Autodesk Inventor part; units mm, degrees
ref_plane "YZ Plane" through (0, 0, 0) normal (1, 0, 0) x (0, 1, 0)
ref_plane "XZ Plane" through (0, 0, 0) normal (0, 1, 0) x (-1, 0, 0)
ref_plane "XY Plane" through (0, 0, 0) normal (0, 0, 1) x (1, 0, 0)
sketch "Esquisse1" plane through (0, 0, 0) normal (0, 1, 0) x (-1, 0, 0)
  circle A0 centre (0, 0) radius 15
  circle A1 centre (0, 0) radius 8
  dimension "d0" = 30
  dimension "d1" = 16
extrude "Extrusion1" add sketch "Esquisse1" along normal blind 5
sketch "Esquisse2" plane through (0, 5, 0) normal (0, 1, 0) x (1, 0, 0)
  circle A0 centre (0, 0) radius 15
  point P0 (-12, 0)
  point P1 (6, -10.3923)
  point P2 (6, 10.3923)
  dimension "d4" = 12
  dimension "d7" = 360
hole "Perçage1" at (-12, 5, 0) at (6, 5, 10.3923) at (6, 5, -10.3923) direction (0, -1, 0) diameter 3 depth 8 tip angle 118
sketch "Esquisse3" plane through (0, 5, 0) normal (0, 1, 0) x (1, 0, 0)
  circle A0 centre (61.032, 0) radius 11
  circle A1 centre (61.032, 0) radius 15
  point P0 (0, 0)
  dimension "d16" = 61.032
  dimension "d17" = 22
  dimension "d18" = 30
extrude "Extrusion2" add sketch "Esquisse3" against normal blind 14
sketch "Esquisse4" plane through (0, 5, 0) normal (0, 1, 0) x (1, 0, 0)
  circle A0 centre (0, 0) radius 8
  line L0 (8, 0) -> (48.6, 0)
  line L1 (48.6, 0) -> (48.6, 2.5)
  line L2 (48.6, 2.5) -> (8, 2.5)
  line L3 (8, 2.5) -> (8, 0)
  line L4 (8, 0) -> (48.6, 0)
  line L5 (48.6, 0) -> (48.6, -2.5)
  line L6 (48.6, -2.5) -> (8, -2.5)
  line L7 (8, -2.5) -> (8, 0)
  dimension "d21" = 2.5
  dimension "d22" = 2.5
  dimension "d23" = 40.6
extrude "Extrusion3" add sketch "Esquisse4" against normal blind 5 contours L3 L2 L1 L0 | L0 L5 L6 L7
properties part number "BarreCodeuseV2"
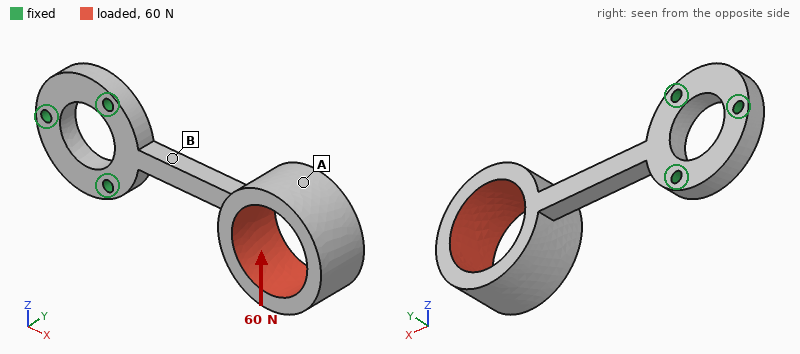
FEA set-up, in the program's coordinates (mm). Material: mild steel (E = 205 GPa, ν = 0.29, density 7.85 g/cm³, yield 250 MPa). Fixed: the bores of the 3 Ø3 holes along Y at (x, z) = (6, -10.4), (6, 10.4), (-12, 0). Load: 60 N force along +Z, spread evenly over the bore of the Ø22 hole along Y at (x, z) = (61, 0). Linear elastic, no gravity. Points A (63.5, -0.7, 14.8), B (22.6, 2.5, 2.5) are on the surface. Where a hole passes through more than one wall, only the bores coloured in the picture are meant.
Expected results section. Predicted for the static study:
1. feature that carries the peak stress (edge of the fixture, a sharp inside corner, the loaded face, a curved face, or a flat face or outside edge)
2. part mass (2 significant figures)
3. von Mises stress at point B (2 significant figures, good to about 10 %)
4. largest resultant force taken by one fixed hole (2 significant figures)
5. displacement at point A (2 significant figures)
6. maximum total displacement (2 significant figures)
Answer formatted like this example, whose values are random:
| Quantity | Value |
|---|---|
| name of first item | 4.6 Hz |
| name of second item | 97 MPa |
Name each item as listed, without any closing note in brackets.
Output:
| Quantity | Value |
|---|---|
| feature that carries the peak stress | a flat face or outside edge |
| part mass | 61 g |
| von Mises stress at point B | 110 MPa |
| largest resultant force taken by one fixed hole | 200 N |
| displacement at point A | 0.25 mm |
| maximum total displacement | 0.32 mm |
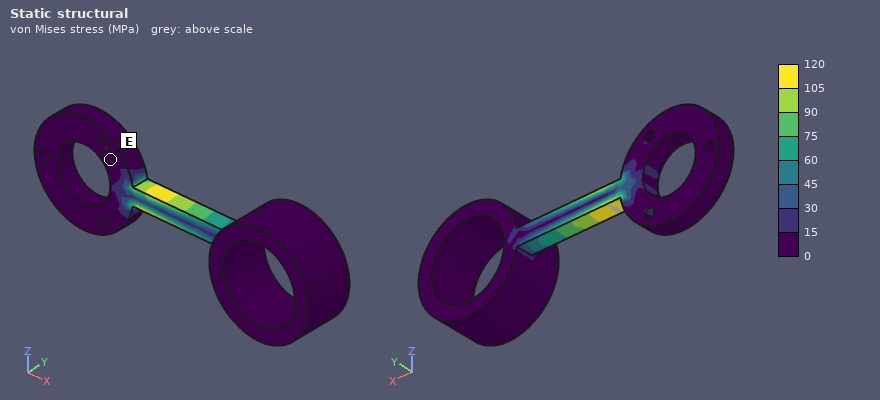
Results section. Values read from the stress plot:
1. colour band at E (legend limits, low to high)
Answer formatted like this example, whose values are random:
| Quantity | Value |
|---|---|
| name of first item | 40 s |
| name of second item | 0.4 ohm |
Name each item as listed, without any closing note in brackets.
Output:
| Quantity | Value |
|---|---|
| colour band at E | 0 to 15 MPa |
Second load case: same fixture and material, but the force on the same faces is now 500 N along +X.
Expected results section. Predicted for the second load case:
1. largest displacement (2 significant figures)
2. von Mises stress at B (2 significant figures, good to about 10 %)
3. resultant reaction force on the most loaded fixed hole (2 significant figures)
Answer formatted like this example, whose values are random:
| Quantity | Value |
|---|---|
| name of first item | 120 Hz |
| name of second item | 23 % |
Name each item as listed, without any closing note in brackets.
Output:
| Quantity | Value |
|---|---|
| largest displacement | 0.41 mm |
| von Mises stress at B | 20 MPa |
| resultant reaction force on the most loaded fixed hole | 330 N |
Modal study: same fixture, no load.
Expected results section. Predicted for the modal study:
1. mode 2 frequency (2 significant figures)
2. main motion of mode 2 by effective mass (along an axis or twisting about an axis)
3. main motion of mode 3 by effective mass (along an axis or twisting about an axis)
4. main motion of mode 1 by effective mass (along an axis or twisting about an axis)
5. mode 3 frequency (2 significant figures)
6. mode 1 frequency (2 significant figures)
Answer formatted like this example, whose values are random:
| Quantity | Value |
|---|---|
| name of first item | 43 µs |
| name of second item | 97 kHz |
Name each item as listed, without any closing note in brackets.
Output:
| Quantity | Value |
|---|---|
| mode 2 frequency | 410 Hz |
| main motion of mode 2 by effective mass | along Z |
| main motion of mode 3 by effective mass | twisting about X |
| main motion of mode 1 by effective mass | along Y |
| mode 3 frequency | 1200 Hz |
| mode 1 frequency | 380 Hz |
